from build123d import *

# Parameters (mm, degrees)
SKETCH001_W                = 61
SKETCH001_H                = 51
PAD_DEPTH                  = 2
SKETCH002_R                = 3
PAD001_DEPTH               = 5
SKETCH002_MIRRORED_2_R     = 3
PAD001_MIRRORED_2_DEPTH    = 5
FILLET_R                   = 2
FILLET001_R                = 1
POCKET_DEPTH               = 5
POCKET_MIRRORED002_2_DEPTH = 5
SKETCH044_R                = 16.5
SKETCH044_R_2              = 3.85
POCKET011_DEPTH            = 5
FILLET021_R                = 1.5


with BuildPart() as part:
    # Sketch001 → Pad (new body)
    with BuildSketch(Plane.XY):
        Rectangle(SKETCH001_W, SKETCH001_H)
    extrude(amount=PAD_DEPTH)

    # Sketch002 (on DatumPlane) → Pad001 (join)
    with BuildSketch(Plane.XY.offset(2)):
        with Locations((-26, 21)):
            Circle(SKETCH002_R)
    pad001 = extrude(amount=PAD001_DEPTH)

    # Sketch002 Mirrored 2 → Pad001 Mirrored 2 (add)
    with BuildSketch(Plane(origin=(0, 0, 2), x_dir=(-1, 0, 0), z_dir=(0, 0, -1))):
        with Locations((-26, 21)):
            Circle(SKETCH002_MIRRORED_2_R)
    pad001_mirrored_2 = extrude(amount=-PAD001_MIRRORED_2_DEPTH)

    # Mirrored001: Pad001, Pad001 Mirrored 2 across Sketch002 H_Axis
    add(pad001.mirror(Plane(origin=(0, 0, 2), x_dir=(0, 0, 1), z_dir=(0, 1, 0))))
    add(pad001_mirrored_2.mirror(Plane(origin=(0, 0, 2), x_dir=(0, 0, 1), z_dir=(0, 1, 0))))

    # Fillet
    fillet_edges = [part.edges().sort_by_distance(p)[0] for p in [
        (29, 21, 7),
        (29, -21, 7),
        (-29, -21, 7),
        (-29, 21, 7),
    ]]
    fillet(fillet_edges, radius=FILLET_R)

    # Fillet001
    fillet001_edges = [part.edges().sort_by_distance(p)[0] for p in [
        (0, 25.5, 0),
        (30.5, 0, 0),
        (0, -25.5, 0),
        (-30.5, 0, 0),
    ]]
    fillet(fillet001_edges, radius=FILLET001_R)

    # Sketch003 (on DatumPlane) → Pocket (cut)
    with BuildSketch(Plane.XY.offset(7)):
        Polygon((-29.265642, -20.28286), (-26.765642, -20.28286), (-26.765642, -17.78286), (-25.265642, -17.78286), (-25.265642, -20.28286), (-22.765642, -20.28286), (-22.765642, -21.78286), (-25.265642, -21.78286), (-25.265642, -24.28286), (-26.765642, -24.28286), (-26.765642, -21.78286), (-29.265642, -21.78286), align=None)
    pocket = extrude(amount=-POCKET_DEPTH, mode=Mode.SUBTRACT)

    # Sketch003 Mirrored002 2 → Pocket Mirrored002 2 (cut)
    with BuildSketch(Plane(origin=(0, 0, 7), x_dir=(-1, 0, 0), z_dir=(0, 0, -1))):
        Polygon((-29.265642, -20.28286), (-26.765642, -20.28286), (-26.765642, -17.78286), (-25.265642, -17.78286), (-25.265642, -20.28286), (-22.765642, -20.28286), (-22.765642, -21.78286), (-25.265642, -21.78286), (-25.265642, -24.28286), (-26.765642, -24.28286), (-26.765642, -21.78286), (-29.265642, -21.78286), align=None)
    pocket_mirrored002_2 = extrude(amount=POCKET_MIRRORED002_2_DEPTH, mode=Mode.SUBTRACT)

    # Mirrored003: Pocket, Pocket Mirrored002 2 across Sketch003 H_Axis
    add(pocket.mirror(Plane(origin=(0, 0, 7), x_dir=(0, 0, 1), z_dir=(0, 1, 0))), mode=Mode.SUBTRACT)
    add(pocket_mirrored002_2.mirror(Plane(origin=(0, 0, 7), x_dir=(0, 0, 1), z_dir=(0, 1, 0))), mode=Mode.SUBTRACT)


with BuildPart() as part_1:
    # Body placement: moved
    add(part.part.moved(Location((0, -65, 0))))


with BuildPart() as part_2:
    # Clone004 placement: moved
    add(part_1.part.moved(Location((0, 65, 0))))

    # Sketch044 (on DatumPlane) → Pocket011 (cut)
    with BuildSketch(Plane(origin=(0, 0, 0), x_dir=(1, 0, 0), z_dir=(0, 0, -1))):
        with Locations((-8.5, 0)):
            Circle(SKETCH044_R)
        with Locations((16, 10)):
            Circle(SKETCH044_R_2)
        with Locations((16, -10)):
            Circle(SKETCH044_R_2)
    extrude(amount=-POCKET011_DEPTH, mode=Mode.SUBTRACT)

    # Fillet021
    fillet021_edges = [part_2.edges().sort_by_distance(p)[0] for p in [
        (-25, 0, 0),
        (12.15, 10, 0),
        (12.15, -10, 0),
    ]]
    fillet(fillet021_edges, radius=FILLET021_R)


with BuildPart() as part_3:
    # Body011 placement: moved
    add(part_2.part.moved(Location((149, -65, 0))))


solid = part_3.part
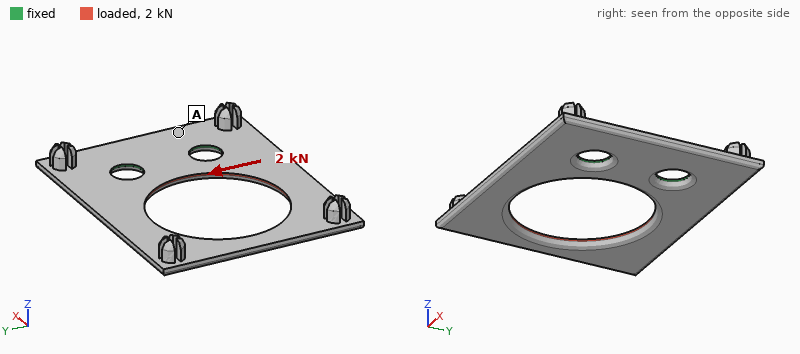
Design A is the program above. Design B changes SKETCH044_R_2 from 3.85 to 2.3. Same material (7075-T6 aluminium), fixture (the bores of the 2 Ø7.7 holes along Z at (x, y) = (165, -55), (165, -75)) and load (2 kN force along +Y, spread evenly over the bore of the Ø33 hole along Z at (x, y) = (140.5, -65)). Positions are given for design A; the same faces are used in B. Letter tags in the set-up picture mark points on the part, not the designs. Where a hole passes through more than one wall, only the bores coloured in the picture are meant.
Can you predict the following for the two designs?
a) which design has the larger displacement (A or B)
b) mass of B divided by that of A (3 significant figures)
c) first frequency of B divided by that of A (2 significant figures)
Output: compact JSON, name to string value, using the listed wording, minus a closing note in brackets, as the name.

{"which design has the larger displacement": "B", "mass of B divided by that of A": "1.03", "first frequency of B divided by that of A": "0.95"}
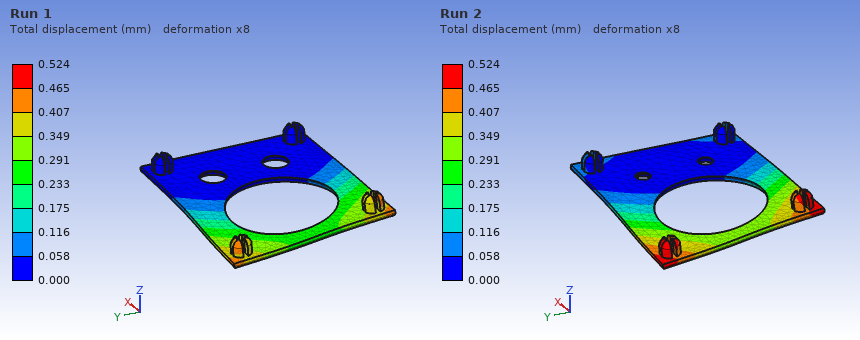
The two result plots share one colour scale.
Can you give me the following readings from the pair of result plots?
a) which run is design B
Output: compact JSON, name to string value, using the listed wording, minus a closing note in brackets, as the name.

{"which run is design B": "Run 2"}
